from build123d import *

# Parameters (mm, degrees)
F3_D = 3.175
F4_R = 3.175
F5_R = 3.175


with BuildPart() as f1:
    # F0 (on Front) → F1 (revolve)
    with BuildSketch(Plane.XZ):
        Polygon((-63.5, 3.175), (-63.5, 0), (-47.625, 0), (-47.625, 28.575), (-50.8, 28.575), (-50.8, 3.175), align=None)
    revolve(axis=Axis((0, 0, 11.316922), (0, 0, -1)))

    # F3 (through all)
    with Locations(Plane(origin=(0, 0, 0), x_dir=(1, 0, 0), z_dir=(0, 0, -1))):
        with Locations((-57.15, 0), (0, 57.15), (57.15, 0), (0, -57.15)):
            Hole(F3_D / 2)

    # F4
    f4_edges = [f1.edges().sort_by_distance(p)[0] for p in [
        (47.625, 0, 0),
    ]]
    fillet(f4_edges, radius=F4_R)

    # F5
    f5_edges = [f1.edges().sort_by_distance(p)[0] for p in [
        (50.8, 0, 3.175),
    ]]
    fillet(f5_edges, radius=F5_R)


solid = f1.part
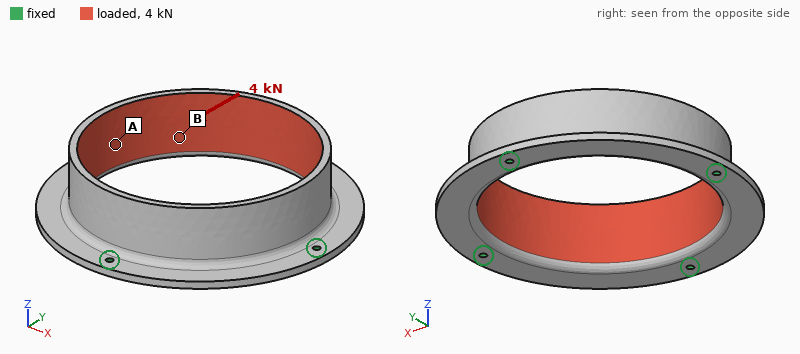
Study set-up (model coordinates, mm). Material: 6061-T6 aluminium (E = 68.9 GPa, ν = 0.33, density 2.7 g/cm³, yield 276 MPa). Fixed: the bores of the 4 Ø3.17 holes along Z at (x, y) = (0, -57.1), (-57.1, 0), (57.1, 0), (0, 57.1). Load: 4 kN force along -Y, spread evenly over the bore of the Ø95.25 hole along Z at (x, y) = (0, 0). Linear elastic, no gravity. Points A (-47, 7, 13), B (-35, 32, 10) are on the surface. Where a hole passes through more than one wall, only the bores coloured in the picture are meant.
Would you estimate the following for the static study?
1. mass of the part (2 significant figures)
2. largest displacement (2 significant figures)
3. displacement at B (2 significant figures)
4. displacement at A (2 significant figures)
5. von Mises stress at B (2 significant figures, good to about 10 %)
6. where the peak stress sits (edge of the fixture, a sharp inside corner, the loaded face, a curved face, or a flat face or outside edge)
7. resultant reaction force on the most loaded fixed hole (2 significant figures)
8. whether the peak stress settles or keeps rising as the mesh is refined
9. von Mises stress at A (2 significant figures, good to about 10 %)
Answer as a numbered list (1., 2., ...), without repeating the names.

1. 110 g
2. 54 µm
3. 26 µm
4. 19 µm
5. 5.3 MPa
6. edge of the fixture
7. 1.4 kN
8. keeps rising
9. 15 MPa
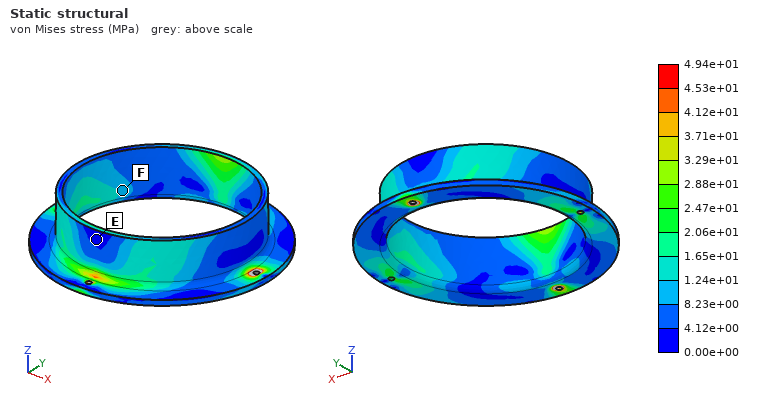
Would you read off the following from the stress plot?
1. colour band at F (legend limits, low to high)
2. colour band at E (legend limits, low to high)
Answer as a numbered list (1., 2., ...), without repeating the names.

1. 8.23e+00 to 1.24e+01 MPa
2. 0.00e+00 to 4.12e+00 MPa
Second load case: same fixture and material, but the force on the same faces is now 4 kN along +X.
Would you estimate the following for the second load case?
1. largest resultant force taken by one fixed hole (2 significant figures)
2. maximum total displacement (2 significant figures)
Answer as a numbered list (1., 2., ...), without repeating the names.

1. 1.4 kN
2. 53 µm
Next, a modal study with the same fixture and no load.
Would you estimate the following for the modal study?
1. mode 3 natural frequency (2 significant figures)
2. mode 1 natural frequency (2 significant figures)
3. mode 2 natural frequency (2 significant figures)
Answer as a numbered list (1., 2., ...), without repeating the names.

1. 3200 Hz
2. 2000 Hz
3. 3200 Hz
